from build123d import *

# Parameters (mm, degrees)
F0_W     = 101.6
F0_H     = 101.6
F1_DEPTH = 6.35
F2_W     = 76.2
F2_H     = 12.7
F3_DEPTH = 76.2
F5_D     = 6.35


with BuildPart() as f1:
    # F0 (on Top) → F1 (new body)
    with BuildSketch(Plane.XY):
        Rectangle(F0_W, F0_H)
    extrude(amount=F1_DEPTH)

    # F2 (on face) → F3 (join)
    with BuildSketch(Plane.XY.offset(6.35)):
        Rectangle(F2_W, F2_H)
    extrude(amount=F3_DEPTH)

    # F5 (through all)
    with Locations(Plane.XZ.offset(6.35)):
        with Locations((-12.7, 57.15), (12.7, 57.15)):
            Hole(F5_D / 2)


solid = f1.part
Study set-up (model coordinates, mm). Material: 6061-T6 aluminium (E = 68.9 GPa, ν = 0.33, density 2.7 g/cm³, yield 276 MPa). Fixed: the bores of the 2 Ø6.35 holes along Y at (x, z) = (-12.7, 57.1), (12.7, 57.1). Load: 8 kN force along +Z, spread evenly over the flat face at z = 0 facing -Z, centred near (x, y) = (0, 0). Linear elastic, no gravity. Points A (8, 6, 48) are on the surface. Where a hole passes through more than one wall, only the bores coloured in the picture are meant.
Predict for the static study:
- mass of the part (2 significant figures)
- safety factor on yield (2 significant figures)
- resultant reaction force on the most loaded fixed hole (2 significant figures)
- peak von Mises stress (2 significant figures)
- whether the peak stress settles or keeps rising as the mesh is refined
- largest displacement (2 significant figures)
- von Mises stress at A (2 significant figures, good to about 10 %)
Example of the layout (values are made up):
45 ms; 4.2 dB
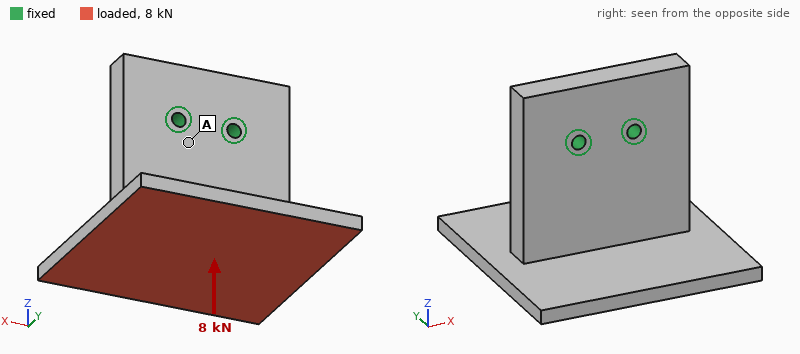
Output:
370 g; 2.6; 4.0 kN; 110 MPa; settles; 0.33 mm; 11 MPa
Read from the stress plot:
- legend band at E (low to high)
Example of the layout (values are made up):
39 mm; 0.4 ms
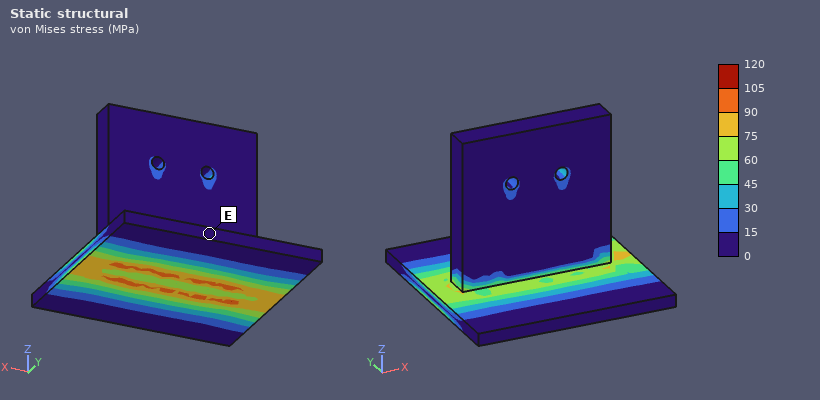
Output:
0 to 15 MPa
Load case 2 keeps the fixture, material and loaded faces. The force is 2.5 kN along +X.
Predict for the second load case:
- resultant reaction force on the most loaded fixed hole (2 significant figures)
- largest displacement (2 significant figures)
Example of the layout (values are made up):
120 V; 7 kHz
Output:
4.9 kN; 39 µm
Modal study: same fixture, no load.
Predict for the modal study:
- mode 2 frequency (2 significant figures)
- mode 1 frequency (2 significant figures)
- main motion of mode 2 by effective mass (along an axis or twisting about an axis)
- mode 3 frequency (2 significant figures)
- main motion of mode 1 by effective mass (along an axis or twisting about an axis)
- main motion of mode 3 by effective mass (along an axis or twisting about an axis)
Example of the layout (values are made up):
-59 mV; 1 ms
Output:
1500 Hz; 1000 Hz; twisting about Z; 2300 Hz; along Y; along Z
